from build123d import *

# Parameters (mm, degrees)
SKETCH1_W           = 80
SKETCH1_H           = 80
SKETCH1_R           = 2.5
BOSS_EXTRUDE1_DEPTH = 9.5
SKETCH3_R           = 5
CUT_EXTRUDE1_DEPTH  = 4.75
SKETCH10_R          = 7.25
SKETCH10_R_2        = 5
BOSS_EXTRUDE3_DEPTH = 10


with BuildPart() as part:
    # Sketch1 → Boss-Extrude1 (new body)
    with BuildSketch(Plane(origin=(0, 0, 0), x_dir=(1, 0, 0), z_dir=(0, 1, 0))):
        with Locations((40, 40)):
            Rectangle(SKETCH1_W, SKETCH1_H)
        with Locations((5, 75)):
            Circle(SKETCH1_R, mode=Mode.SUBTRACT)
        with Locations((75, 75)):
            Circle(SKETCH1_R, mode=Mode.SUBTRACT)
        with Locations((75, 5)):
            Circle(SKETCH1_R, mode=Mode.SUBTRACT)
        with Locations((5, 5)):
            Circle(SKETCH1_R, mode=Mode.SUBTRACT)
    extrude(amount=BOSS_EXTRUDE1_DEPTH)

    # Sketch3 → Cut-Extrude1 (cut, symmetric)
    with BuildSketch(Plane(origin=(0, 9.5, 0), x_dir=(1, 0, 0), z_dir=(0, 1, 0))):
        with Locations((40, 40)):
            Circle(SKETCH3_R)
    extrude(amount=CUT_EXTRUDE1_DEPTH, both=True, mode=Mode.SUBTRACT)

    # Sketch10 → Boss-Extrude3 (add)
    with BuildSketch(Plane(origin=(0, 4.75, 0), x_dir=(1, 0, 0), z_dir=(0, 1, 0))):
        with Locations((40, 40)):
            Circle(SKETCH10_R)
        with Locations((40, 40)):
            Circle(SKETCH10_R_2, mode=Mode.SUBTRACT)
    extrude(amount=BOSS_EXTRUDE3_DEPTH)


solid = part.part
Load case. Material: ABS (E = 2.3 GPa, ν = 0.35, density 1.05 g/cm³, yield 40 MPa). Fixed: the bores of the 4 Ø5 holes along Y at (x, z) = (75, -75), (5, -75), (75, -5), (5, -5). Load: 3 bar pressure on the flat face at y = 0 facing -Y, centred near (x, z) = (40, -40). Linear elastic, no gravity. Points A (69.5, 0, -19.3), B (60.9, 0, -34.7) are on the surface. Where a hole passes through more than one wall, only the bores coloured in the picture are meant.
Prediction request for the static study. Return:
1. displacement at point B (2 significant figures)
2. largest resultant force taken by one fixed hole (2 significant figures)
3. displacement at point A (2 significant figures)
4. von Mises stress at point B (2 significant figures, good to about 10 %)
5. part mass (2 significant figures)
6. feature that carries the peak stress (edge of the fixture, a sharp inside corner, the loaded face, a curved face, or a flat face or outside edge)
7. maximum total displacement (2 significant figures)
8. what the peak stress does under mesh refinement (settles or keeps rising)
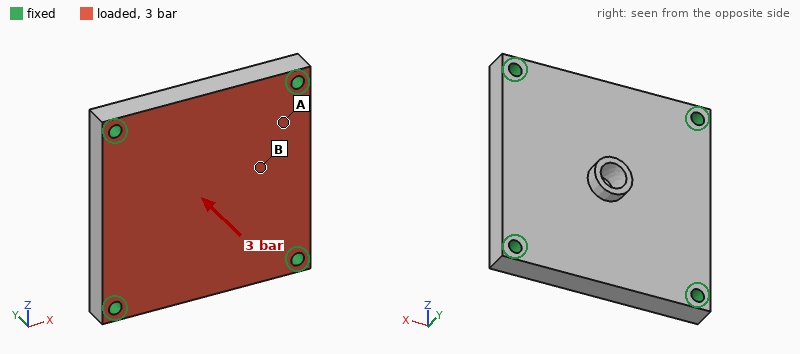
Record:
0.30 mm
470 N
0.15 mm
4.8 MPa
63 g
edge of the fixture
0.38 mm
keeps rising
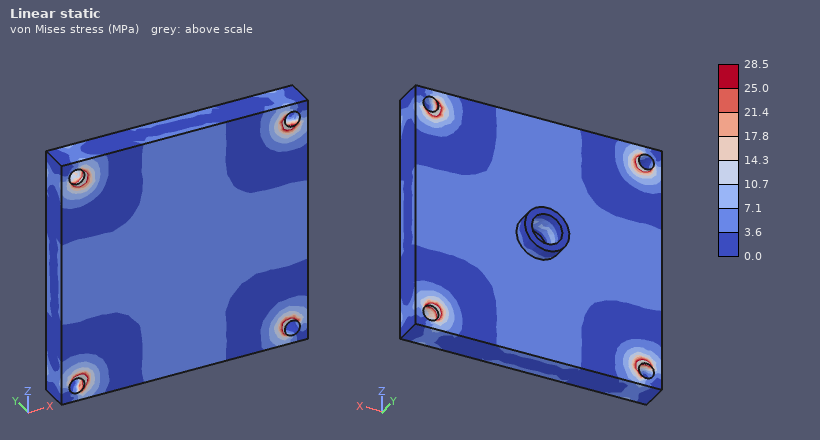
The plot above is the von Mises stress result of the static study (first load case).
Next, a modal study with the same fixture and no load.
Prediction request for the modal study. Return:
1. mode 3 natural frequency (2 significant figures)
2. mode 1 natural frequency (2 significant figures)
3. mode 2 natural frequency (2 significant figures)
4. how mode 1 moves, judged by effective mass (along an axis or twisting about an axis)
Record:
2800 Hz
1700 Hz
2800 Hz
along Y
